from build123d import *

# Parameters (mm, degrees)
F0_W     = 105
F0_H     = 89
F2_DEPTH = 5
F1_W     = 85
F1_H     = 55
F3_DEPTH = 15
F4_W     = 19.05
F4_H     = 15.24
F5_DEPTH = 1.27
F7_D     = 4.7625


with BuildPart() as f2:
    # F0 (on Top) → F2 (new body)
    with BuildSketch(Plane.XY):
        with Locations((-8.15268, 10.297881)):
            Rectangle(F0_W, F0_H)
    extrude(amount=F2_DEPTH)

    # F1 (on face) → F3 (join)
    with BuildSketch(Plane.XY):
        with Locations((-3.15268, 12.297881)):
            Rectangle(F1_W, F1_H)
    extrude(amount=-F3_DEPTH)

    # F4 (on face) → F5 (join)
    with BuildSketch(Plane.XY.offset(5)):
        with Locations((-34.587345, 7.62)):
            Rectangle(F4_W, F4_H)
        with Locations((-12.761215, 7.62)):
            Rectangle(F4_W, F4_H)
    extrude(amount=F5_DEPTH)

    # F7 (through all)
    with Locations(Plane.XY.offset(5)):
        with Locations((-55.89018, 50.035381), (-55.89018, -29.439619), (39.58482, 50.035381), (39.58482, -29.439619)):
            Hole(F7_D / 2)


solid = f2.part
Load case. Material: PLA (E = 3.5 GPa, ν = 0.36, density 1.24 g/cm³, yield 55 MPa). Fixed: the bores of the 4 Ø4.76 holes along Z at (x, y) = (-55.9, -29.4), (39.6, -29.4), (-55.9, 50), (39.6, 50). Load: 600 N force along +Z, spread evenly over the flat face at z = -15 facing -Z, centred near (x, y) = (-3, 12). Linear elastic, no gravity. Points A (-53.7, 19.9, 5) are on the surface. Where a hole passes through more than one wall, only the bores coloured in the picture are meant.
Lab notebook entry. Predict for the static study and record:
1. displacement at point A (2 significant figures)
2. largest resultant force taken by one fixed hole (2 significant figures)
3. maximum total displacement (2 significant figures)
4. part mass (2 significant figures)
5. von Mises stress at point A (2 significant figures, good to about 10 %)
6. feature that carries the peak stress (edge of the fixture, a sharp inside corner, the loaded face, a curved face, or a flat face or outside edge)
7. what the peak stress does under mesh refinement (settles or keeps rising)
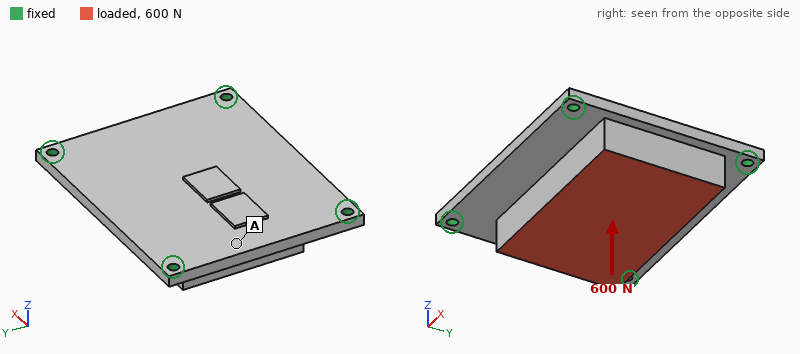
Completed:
0.14 mm
210 N
0.17 mm
150 g
2.4 MPa
edge of the fixture
keeps rising
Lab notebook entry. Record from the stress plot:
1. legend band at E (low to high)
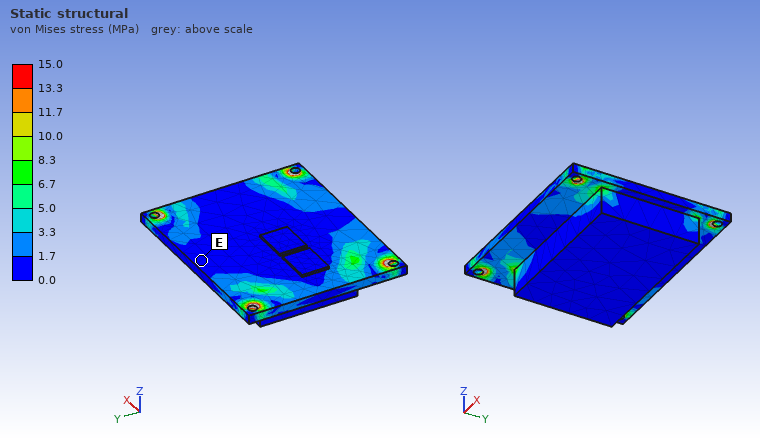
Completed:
0.0 to 1.7 MPa
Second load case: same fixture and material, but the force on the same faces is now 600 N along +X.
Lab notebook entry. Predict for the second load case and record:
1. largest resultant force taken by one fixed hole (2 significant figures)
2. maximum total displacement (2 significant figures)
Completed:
200 N
75 µm
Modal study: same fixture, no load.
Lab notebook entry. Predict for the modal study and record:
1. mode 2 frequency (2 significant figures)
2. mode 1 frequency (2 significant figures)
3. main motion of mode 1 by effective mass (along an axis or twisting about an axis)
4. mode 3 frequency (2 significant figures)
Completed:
1500 Hz
870 Hz
along Z
1600 Hz
